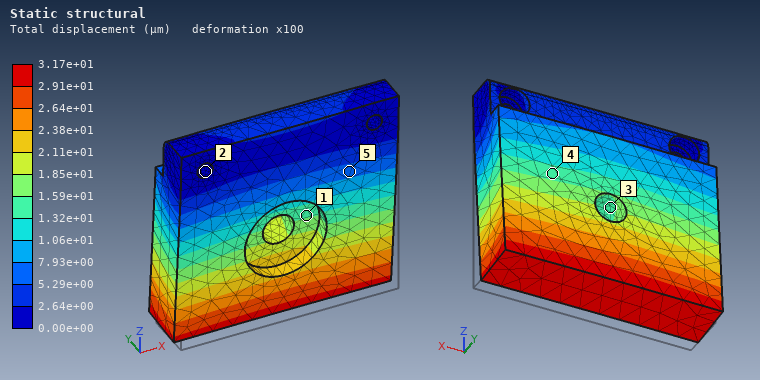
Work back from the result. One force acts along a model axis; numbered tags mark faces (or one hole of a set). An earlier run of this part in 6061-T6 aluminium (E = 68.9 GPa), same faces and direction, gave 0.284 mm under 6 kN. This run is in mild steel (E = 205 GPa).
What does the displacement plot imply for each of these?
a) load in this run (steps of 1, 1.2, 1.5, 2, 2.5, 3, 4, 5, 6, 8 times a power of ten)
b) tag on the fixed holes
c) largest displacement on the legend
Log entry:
2 kN
2
3.17e+01 µm
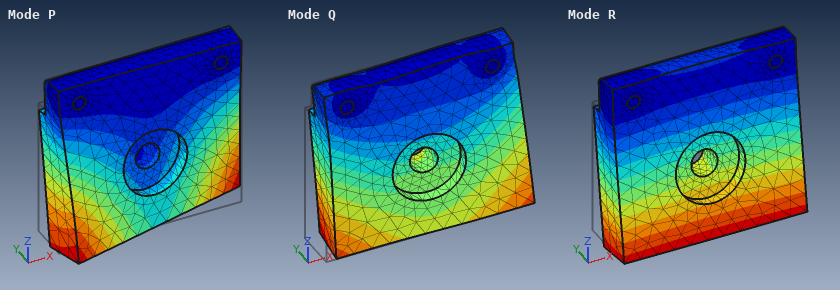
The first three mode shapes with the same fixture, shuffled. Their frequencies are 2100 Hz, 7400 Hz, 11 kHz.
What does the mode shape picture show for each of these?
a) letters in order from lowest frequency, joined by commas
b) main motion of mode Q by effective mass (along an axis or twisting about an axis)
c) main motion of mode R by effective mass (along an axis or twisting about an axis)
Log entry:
R, P, Q
along X
along Y
